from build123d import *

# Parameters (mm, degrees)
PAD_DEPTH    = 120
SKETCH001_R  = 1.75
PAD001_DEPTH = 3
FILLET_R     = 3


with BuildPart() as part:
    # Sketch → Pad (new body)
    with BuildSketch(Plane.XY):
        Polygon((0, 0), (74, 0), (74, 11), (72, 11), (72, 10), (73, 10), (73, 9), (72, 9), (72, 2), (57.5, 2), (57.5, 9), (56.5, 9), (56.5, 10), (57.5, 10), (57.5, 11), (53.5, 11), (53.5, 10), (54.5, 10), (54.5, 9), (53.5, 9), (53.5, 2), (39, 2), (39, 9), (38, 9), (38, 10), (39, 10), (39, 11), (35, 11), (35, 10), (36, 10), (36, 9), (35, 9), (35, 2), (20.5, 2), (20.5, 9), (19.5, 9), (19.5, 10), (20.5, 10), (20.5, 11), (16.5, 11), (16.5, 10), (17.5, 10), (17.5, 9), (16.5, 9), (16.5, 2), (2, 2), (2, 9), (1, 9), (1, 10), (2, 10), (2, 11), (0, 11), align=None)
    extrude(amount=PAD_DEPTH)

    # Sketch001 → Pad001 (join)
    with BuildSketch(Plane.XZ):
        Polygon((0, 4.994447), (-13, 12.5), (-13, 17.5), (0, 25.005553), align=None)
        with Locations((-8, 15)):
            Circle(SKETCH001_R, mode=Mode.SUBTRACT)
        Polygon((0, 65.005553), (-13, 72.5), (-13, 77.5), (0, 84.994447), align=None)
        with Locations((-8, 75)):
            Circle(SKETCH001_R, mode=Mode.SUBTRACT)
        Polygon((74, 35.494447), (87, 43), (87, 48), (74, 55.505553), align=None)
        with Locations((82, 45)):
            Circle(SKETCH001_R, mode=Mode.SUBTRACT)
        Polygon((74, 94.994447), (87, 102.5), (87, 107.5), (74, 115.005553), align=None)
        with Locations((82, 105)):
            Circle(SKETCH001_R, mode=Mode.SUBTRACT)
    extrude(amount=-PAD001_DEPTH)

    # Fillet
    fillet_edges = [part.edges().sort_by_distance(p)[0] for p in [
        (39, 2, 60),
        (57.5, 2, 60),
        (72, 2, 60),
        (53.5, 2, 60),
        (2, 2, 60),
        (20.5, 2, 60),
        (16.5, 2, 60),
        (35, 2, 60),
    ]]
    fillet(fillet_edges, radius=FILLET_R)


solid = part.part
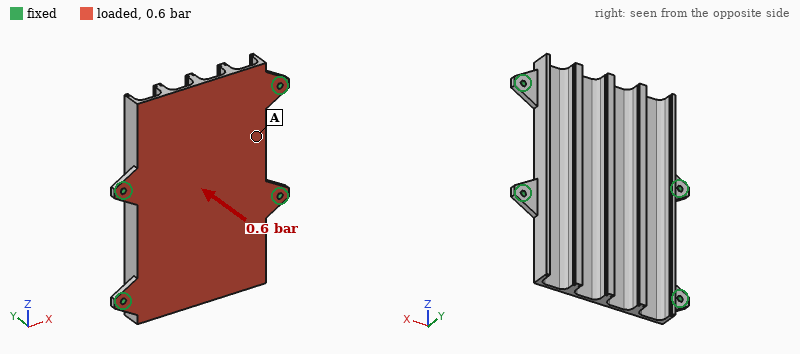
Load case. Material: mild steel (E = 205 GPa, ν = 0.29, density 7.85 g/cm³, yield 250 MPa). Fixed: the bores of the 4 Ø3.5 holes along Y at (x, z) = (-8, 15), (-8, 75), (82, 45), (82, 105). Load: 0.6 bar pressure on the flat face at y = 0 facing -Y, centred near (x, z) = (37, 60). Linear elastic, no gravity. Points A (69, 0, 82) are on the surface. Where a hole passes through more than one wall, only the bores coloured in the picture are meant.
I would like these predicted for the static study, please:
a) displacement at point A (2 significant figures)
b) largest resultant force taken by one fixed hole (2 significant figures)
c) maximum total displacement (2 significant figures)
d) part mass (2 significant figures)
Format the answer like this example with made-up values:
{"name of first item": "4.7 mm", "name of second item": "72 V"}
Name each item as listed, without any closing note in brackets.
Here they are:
{"displacement at point A": "18 µm", "largest resultant force taken by one fixed hole": "300 N", "maximum total displacement": "68 µm", "part mass": "300 g"}
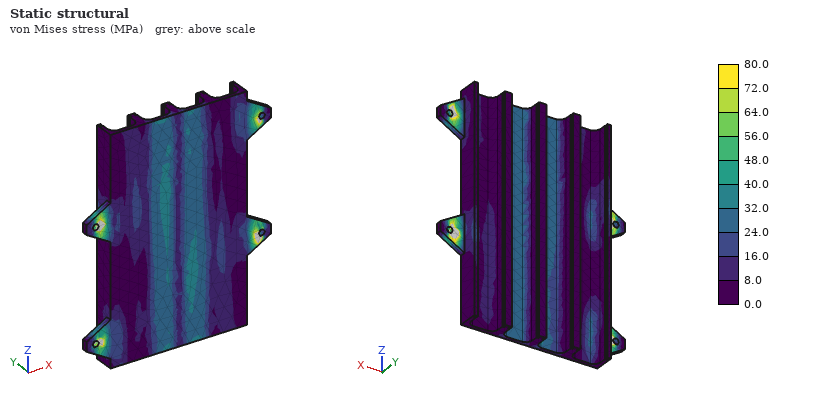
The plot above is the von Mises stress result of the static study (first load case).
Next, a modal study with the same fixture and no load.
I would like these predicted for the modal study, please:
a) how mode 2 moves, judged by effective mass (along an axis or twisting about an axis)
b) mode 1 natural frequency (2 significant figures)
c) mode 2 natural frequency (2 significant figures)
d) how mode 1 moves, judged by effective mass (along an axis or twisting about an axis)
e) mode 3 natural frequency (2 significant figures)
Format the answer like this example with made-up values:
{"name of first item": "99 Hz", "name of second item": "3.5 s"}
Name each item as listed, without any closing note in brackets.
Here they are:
{"how mode 2 moves, judged by effective mass": "twisting about X", "mode 1 natural frequency": "960 Hz", "mode 2 natural frequency": "1200 Hz", "how mode 1 moves, judged by effective mass": "along Y", "mode 3 natural frequency": "2600 Hz"}
